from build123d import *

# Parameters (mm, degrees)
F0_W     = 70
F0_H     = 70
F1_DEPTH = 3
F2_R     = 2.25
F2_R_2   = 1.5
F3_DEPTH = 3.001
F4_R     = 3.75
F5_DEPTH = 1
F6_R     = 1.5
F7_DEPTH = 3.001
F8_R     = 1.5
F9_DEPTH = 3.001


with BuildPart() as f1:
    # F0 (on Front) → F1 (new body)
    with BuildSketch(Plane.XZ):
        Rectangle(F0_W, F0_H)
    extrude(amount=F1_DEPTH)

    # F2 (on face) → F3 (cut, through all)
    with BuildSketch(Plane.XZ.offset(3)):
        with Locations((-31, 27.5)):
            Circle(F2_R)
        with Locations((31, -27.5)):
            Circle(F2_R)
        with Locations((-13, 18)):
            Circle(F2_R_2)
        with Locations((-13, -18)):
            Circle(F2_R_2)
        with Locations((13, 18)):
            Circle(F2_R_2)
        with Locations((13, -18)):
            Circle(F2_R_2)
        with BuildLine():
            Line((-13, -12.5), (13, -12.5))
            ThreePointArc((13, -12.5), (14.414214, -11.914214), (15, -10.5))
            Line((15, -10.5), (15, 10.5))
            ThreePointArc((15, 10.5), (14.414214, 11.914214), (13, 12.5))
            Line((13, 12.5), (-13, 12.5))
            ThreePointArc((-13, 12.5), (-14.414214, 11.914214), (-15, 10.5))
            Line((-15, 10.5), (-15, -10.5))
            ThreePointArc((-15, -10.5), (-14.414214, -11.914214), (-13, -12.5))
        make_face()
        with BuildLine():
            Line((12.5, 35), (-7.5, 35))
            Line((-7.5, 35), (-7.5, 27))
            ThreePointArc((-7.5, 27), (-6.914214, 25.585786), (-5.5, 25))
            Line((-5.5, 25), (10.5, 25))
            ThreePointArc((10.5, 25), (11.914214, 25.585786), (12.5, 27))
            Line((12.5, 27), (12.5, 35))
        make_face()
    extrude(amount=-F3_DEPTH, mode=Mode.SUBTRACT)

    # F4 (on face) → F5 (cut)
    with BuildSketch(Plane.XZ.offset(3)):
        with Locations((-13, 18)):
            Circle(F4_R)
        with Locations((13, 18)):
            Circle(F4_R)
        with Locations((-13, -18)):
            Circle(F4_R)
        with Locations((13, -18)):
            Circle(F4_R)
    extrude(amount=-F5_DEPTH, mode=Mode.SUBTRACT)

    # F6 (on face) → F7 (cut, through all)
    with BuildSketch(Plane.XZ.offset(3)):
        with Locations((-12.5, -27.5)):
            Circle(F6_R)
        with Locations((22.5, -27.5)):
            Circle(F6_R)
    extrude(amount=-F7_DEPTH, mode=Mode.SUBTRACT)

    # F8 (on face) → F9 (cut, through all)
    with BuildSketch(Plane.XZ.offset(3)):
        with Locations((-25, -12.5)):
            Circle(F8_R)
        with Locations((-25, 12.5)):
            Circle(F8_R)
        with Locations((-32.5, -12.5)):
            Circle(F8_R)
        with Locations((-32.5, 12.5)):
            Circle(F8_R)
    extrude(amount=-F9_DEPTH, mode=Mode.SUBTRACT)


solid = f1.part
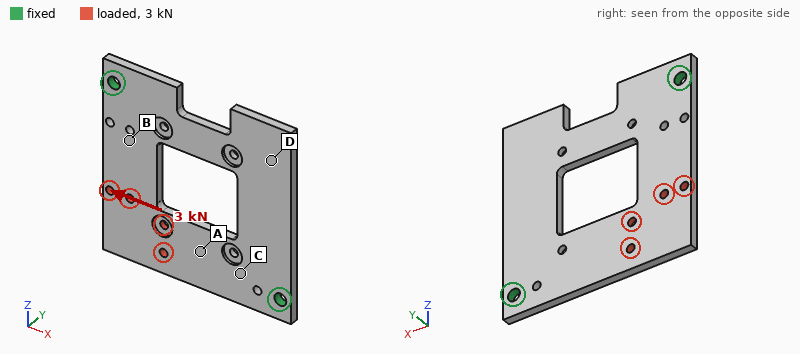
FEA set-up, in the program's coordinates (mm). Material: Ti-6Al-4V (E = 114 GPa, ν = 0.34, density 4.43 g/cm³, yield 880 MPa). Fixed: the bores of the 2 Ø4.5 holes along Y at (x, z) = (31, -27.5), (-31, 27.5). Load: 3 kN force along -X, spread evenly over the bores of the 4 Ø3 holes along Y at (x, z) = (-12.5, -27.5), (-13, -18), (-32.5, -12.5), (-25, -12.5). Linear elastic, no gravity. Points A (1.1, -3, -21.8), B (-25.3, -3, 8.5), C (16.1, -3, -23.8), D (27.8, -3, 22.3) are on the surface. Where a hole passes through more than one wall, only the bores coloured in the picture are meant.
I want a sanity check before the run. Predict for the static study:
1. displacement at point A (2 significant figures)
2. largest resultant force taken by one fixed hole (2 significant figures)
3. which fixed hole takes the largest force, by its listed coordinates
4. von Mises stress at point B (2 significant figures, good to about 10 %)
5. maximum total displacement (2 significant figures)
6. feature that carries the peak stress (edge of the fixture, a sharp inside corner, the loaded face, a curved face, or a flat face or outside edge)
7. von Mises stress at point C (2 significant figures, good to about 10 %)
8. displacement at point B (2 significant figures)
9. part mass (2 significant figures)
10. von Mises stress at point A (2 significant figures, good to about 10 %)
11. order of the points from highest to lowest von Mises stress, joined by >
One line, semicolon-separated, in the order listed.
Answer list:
14 µm; 2.4 kN; (31, -27.5); 19 MPa; 29 µm; a curved face; 50 MPa; 13 µm; 51 g; 33 MPa; C > A > B > D
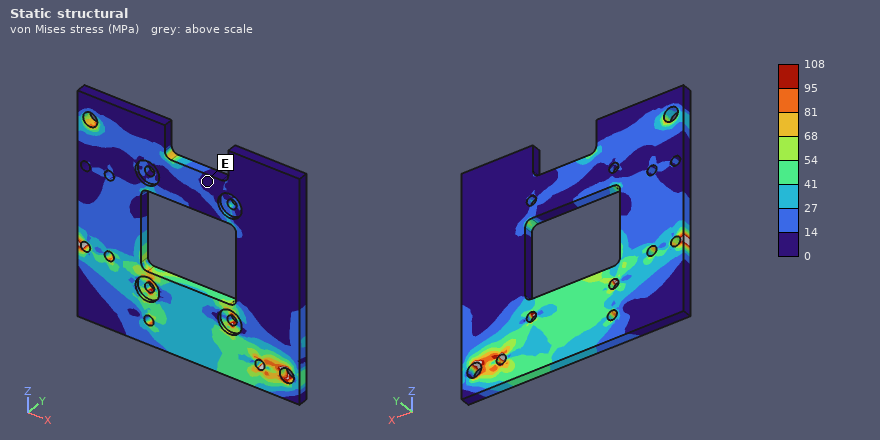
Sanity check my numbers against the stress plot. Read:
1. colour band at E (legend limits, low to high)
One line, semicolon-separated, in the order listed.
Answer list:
0 to 14 MPa
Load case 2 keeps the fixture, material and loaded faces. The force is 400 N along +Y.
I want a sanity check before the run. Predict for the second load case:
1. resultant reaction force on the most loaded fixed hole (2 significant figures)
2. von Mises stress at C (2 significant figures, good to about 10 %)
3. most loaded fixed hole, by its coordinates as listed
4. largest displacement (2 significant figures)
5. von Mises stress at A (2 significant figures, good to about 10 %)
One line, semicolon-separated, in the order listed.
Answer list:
230 N; 140 MPa; (-31, 27.5); 1.1 mm; 63 MPa
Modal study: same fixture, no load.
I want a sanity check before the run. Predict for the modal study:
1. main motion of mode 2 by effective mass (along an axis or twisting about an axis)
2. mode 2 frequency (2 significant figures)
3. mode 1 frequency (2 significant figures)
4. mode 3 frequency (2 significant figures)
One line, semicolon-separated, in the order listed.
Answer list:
along Y; 1100 Hz; 900 Hz; 3200 Hz
